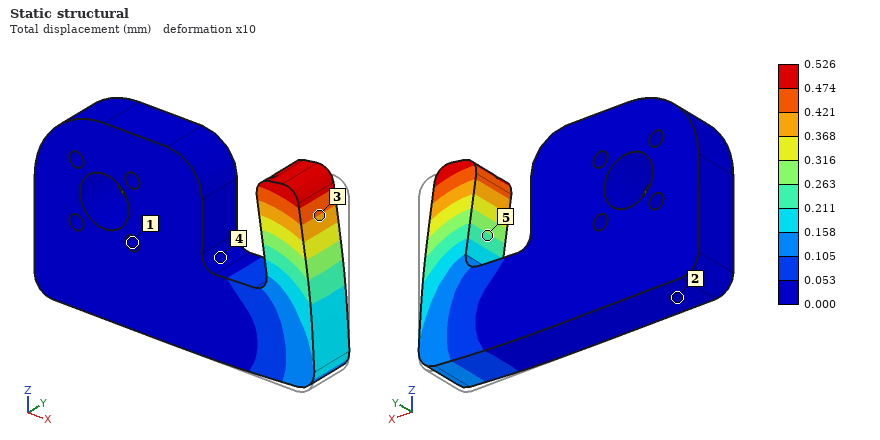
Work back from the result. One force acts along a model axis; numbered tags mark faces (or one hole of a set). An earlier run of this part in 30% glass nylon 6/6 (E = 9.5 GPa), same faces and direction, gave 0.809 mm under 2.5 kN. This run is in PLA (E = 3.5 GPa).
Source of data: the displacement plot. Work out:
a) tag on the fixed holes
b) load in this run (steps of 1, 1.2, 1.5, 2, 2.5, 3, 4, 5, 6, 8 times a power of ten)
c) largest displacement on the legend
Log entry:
1
600 N
0.526 mm
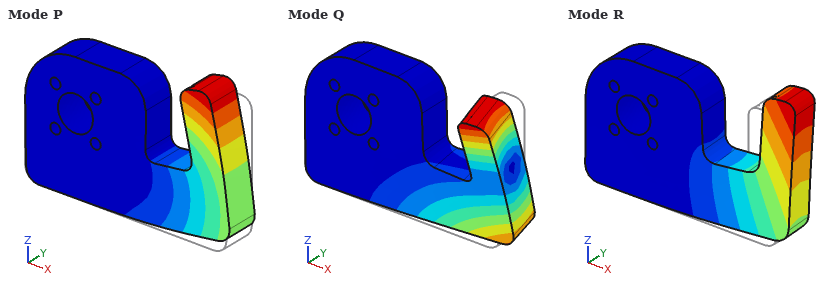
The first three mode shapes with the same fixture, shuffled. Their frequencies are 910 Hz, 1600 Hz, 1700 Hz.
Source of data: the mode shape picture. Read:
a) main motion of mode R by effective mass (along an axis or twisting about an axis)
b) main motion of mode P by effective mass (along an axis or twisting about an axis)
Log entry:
along Y
along Z
